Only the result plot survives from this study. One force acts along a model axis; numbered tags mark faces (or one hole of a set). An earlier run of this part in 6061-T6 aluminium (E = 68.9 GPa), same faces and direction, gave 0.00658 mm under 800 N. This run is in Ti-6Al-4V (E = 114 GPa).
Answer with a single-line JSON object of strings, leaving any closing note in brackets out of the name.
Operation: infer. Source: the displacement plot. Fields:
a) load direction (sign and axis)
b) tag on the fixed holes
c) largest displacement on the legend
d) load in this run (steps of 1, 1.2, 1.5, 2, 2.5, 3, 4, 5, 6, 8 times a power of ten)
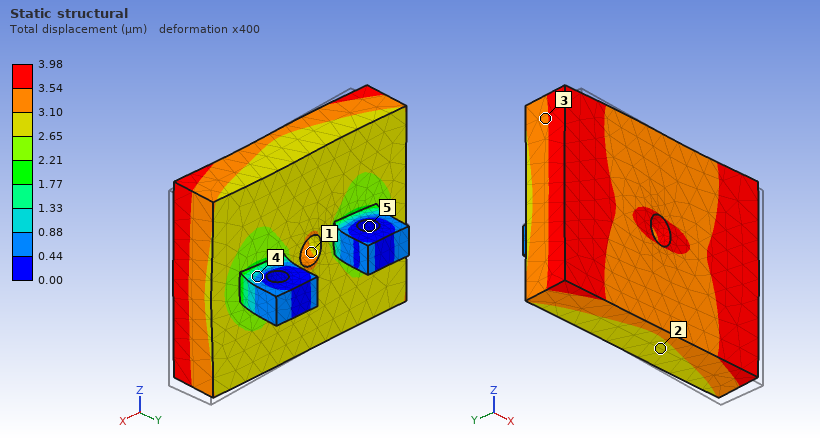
{"load direction": "-X", "tag on the fixed holes": "5", "largest displacement on the legend": "3.98 µm", "load in this run": "800 N"}
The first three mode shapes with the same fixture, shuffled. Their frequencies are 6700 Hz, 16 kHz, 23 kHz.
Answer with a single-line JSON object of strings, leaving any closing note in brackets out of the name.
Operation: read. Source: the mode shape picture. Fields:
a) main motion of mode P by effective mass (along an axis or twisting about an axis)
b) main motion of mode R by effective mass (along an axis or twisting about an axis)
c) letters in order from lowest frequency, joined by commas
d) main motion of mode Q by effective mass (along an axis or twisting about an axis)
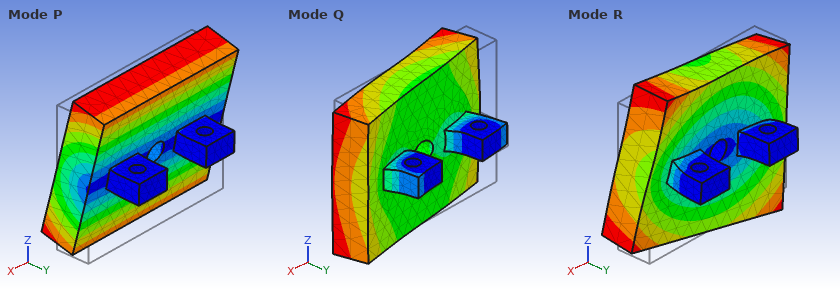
{"main motion of mode P by effective mass": "along Z", "main motion of mode R by effective mass": "twisting about Y", "letters in order from lowest frequency, joined by commas": "P, R, Q", "main motion of mode Q by effective mass": "along X"}
